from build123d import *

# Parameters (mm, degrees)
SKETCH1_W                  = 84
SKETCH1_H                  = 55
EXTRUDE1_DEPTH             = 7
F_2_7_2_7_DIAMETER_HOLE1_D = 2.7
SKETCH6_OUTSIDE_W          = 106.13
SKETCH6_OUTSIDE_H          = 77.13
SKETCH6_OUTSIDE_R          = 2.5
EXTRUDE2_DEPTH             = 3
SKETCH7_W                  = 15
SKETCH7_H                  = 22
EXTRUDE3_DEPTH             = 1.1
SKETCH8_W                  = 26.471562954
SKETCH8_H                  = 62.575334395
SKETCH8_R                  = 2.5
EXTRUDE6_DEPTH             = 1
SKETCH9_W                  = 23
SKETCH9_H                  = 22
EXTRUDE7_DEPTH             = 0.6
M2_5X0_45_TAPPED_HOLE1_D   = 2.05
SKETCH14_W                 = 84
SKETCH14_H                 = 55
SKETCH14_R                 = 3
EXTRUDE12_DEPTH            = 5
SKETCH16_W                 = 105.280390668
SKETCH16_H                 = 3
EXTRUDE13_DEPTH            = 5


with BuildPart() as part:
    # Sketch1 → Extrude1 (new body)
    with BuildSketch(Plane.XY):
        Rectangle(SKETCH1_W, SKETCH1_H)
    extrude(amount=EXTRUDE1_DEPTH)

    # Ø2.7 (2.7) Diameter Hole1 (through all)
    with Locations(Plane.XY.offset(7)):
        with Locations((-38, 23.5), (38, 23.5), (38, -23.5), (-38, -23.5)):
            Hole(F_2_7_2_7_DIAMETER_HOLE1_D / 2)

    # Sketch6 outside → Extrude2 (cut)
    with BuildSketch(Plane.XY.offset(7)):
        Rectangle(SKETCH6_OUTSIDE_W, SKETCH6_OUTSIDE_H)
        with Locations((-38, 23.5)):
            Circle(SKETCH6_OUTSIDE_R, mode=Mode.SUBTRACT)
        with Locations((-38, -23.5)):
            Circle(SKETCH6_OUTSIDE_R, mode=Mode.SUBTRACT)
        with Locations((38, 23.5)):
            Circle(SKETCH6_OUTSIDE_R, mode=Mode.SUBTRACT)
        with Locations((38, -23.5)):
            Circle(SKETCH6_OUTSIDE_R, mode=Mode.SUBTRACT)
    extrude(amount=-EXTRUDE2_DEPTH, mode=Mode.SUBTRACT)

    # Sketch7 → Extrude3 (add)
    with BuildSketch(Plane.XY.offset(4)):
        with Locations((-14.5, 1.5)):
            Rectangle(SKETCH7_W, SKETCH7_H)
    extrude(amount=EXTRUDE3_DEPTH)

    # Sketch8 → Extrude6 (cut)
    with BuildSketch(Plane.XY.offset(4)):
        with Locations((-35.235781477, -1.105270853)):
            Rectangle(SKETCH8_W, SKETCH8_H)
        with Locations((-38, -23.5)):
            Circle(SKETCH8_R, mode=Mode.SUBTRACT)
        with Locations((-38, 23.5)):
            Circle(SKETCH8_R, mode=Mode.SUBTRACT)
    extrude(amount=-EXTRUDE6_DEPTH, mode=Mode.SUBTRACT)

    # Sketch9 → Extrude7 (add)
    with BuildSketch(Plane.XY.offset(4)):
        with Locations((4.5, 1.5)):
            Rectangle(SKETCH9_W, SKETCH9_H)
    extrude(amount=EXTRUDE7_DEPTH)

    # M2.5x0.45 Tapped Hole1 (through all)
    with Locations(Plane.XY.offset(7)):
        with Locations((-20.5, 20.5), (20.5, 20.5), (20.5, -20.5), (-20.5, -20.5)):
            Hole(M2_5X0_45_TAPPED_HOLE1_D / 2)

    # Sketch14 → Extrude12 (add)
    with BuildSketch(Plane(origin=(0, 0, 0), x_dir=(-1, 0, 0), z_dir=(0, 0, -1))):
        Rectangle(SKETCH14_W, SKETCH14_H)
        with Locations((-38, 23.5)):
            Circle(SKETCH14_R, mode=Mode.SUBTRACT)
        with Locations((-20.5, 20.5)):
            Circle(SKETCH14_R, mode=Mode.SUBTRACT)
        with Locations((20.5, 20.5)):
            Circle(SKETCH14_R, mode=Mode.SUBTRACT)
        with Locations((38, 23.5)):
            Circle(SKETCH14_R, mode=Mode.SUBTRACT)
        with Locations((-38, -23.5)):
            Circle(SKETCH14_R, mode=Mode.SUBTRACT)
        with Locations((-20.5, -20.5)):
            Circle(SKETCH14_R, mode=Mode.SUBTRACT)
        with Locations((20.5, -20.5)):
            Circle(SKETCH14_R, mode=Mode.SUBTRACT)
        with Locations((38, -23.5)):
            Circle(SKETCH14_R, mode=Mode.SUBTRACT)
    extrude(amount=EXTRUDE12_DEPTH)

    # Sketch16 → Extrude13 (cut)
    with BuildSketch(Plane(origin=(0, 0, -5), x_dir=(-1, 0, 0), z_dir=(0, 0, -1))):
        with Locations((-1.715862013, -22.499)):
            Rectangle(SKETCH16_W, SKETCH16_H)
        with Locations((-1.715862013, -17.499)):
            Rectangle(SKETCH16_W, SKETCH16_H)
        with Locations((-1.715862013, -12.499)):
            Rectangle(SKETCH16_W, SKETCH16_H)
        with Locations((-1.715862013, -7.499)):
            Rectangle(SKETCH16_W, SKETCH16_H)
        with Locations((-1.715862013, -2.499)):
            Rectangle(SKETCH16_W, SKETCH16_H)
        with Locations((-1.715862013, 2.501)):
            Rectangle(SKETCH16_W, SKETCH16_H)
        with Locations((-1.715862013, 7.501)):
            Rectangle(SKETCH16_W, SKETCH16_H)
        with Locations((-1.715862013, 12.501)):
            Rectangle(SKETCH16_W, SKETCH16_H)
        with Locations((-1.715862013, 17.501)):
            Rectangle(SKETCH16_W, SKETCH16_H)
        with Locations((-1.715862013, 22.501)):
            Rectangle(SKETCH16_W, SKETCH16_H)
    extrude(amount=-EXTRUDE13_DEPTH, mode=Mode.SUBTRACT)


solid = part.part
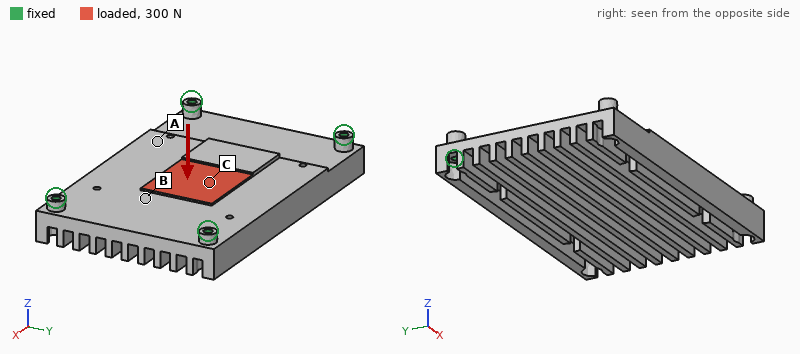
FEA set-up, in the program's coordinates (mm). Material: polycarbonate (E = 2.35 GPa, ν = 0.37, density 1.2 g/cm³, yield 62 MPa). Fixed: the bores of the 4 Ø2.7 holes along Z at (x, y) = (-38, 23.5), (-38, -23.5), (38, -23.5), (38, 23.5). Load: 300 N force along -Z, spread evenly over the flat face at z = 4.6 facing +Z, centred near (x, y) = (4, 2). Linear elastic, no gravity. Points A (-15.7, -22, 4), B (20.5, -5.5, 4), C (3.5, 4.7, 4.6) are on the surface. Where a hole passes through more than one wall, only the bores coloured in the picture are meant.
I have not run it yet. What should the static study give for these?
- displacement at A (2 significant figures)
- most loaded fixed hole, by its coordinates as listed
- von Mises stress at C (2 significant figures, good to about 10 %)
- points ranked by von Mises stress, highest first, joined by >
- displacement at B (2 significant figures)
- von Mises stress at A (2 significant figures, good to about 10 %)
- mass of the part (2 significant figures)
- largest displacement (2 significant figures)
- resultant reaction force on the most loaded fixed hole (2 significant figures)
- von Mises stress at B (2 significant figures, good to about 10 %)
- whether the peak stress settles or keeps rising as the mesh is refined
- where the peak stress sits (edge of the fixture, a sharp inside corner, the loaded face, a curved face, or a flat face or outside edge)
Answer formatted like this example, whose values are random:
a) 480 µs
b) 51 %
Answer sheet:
a) 0.22 mm
b) (38, 23.5)
c) 8.3 MPa
d) C > B > A
e) 0.38 mm
f) 2.4 MPa
g) 34 g
h) 0.51 mm
i) 110 N
j) 5.3 MPa
k) keeps rising
l) edge of the fixture
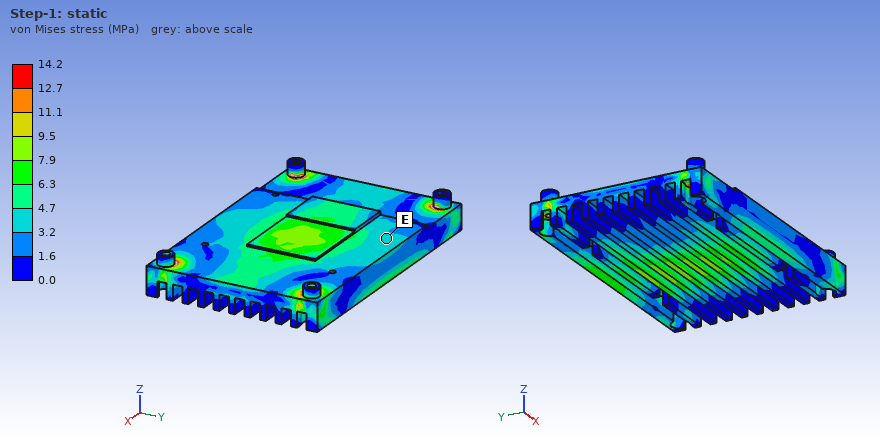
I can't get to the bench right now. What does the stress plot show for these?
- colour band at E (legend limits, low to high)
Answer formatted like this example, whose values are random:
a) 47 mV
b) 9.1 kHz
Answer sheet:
a) 3.2 to 4.7 MPa
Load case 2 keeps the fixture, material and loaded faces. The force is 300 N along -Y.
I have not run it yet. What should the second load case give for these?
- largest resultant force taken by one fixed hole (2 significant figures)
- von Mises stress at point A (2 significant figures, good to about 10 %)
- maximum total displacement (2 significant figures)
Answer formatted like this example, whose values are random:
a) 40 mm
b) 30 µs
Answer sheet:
a) 100 N
b) 0.75 MPa
c) 51 µm
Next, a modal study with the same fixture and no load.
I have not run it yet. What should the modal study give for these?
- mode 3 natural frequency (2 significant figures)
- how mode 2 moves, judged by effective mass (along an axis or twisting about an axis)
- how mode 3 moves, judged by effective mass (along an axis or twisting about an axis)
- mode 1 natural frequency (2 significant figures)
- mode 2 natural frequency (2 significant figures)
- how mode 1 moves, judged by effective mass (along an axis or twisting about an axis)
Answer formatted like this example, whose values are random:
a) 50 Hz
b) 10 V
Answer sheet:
a) 1800 Hz
b) twisting about X
c) twisting about Y
d) 1000 Hz
e) 1500 Hz
f) along Z
